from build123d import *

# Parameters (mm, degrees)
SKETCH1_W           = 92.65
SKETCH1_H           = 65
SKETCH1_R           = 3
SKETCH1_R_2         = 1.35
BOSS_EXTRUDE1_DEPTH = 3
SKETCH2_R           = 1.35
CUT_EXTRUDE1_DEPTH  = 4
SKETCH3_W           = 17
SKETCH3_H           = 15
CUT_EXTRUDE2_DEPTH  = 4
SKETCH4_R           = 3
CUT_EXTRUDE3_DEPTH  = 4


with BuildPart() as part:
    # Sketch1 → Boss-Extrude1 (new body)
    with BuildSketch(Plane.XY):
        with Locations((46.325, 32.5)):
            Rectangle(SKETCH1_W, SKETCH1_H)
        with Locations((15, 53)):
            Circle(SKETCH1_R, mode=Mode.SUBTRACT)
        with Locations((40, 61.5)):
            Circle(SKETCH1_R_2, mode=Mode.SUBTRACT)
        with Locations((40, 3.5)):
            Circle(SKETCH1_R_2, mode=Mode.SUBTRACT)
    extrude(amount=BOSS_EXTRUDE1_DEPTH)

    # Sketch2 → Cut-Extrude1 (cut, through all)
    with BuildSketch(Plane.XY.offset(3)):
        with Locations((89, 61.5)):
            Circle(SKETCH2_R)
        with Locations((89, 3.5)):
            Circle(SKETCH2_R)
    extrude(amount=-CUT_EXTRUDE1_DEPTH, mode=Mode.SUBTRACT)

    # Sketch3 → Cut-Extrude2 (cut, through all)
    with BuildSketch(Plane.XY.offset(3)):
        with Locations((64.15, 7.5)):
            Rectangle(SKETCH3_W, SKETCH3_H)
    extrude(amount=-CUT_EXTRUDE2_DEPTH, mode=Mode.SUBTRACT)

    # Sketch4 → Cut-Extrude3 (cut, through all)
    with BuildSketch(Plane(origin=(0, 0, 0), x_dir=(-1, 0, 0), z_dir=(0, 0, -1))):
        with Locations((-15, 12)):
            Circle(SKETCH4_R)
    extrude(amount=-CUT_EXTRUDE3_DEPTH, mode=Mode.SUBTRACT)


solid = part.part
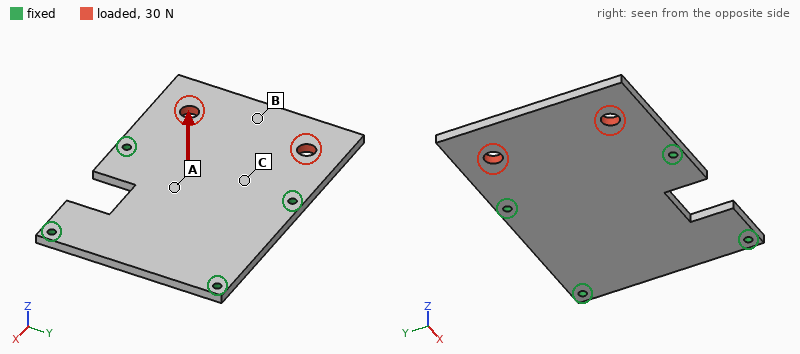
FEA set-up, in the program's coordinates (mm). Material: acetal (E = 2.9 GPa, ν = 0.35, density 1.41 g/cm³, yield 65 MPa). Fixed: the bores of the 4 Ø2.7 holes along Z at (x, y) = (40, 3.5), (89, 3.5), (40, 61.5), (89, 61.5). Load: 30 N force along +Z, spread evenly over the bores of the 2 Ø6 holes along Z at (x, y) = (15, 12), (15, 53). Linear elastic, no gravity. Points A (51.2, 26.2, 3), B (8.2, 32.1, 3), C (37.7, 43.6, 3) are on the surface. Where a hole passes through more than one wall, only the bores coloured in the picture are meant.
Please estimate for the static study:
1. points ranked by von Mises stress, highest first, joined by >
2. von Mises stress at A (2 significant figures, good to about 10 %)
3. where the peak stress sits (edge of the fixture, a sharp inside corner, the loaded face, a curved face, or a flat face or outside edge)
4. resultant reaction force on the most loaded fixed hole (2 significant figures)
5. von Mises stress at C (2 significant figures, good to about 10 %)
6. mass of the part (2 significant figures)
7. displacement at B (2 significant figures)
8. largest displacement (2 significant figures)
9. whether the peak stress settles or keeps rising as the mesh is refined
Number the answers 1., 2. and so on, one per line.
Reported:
1. C > A > B
2. 2.3 MPa
3. edge of the fixture
4. 18 N
5. 4.2 MPa
6. 24 g
7. 0.86 mm
8. 1.1 mm
9. keeps rising
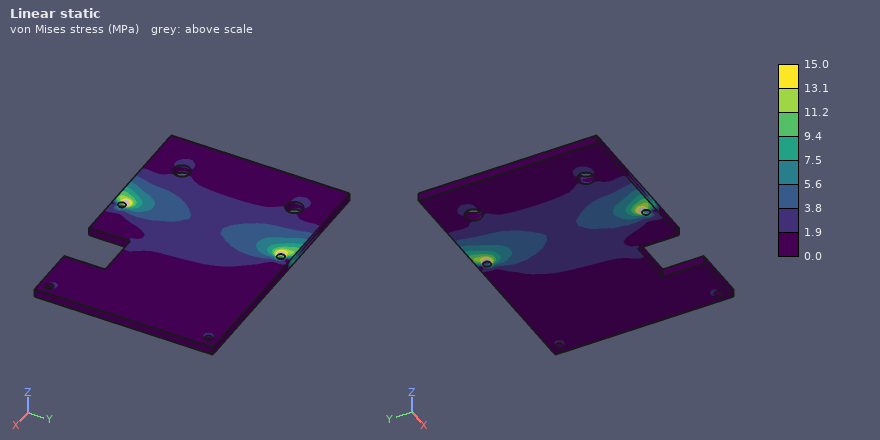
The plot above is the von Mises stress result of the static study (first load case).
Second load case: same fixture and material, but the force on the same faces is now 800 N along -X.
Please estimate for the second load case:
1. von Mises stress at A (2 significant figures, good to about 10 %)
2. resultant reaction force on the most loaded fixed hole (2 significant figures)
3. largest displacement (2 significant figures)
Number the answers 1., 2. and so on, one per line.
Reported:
1. 2.2 MPa
2. 330 N
3. 84 µm
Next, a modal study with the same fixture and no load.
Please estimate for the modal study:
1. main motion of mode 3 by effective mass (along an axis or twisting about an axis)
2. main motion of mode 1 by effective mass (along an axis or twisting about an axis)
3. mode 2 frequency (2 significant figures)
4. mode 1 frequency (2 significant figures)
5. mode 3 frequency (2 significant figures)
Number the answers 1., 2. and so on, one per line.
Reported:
1. along Z
2. along Z
3. 740 Hz
4. 350 Hz
5. 950 Hz
